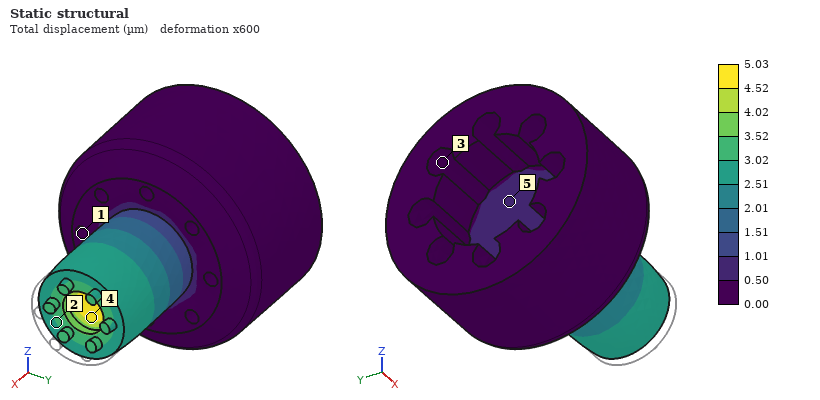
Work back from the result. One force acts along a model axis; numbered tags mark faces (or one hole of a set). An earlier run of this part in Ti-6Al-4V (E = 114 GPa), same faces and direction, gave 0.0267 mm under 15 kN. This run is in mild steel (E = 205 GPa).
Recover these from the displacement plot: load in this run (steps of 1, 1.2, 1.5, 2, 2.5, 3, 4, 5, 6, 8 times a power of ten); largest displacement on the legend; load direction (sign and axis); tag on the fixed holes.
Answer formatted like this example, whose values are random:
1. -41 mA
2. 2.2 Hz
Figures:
1. 5 kN
2. 5.03 µm
3. -X
4. 1
